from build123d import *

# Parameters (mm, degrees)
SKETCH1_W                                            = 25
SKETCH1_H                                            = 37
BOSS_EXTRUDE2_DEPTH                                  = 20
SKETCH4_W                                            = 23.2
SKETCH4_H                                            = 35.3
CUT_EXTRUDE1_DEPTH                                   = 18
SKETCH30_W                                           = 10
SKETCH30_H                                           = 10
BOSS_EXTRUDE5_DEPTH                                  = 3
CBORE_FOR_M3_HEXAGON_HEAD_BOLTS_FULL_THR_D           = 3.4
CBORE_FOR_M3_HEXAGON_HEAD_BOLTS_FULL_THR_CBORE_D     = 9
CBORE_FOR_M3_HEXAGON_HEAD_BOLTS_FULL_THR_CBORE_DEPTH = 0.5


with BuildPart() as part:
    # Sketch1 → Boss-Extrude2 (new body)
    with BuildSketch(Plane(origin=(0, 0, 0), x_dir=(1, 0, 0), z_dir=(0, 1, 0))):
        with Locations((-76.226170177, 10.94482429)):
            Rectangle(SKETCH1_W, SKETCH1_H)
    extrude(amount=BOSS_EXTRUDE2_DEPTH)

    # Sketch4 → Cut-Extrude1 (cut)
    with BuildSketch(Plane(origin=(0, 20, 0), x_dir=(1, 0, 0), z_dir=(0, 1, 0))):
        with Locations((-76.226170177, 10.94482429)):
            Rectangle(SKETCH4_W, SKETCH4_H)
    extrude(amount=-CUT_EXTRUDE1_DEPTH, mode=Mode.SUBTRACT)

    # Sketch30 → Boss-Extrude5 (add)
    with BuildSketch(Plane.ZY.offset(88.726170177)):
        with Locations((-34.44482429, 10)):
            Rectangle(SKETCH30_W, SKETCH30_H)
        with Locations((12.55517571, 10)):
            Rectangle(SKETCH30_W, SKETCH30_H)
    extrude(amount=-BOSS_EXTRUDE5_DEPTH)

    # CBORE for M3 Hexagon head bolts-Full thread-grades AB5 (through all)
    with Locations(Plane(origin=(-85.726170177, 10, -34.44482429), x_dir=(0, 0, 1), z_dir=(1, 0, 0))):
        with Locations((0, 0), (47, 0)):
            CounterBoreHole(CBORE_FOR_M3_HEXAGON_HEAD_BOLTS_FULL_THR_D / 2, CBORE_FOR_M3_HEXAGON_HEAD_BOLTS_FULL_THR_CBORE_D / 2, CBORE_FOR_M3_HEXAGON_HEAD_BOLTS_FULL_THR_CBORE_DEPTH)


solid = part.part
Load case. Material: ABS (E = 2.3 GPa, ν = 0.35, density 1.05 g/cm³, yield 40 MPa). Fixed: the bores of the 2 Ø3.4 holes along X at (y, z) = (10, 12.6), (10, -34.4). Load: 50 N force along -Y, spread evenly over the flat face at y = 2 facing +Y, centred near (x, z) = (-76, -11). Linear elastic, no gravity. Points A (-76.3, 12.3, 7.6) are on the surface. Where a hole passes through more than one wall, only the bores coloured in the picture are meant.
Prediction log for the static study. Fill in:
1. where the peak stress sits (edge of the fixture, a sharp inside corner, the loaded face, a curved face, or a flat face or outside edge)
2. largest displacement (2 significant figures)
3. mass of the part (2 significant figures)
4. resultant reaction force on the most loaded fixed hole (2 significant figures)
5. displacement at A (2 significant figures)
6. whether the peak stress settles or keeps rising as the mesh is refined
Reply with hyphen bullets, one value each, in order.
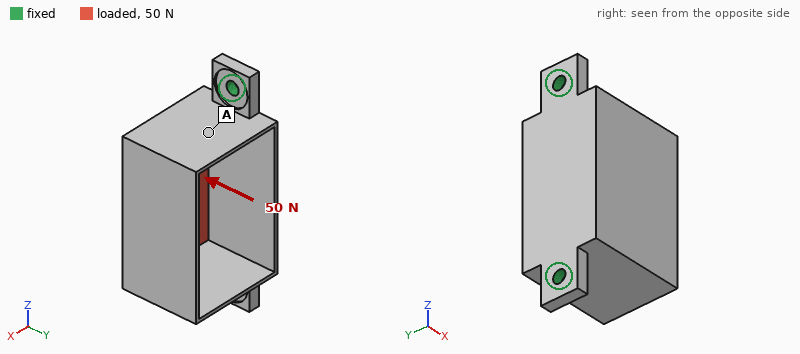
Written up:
- edge of the fixture
- 0.71 mm
- 4.5 g
- 25 N
- 0.31 mm
- keeps rising
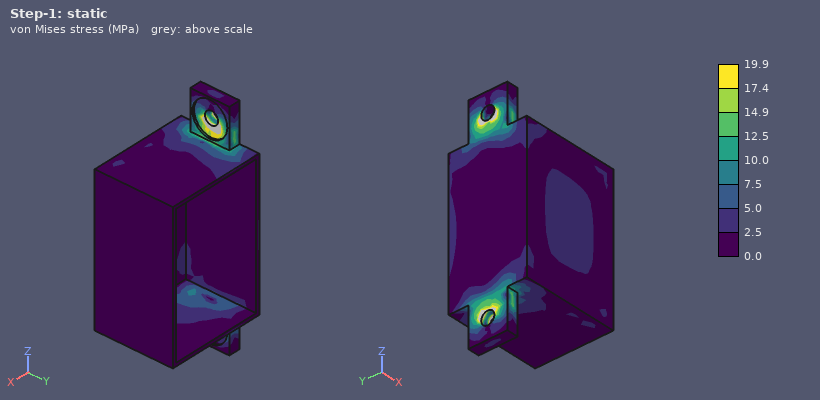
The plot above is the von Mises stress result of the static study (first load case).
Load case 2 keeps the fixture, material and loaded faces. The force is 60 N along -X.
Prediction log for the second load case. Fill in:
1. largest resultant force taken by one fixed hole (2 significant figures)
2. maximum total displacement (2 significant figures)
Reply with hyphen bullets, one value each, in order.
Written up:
- 30 N
- 0.60 mm
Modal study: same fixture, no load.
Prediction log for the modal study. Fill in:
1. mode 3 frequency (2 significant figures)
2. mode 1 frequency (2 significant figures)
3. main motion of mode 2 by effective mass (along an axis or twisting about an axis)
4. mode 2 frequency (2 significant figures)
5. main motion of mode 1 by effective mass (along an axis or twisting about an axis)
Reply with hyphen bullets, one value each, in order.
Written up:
- 1200 Hz
- 710 Hz
- along Z
- 840 Hz
- along Y
